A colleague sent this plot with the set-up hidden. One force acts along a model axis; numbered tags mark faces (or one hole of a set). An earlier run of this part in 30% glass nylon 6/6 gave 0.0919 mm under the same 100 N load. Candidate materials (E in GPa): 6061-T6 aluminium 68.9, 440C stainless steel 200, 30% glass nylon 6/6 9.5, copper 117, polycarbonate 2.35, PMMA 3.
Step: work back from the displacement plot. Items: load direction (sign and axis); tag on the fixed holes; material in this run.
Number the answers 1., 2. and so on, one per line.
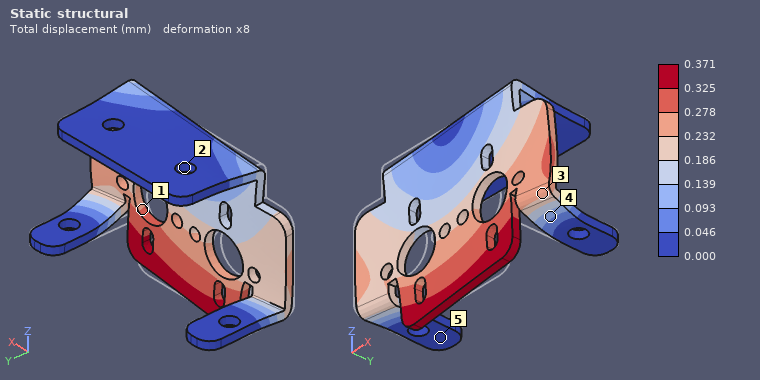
1. +X
2. 2
3. polycarbonate
